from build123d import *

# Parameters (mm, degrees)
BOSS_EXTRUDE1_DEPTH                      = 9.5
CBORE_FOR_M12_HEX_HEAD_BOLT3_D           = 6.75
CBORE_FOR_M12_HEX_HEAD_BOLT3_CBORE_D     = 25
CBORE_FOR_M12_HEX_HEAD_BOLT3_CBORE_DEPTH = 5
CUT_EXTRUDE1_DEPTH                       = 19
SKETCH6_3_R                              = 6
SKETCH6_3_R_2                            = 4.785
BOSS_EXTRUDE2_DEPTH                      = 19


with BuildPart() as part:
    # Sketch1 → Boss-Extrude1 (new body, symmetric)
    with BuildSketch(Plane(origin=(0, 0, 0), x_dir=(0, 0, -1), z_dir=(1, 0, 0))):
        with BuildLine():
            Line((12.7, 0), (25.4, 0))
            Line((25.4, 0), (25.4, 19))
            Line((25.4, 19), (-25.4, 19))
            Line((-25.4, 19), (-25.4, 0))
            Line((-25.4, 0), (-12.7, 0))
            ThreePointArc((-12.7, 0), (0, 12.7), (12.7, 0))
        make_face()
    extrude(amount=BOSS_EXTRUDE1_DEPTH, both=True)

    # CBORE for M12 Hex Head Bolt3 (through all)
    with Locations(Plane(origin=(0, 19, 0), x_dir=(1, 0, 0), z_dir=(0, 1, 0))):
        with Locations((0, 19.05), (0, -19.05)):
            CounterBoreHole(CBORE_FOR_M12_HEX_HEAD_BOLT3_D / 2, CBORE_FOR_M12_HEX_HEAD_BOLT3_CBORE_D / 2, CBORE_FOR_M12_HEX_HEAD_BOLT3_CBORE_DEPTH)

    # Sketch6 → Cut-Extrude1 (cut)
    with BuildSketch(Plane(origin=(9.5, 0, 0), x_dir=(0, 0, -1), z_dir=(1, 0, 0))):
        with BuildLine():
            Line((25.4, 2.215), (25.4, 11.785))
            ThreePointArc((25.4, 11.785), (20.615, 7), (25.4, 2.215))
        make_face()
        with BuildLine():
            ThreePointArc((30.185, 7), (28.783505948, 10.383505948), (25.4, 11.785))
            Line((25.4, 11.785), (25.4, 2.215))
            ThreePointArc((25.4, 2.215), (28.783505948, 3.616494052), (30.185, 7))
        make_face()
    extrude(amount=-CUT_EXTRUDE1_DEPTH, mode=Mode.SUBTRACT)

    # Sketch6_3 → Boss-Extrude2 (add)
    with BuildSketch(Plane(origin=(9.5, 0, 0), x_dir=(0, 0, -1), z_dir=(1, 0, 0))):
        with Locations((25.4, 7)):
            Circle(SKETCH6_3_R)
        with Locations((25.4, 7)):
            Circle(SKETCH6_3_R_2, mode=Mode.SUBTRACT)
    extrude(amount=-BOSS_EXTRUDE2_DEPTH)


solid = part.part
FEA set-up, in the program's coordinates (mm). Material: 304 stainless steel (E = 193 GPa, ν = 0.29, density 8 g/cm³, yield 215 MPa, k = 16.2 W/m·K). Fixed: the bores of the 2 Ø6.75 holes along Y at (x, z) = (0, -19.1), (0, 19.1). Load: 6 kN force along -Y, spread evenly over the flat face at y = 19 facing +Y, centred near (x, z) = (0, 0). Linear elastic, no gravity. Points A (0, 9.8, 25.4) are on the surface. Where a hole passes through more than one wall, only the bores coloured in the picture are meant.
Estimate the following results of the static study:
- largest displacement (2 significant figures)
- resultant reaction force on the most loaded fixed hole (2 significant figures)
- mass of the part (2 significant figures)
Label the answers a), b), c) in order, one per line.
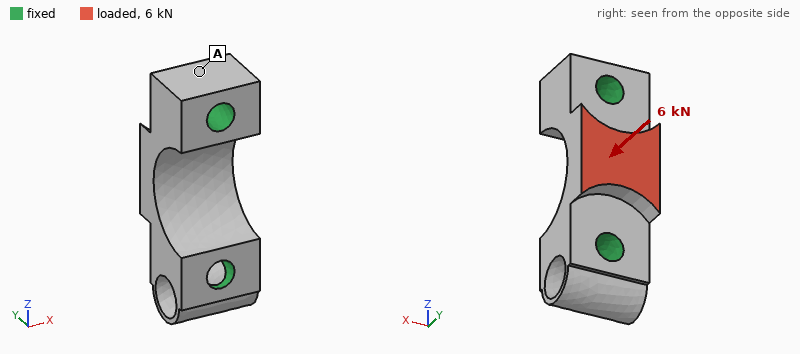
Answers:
a) 7.7 µm
b) 3.9 kN
c) 72 g
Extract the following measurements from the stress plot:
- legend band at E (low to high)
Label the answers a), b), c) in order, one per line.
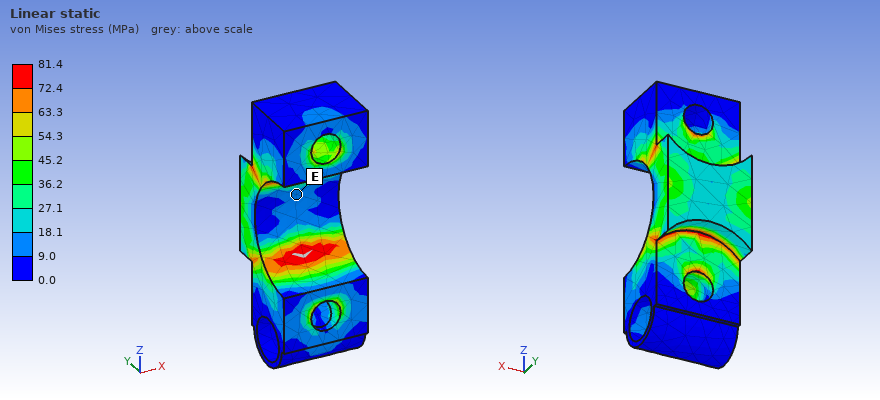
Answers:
a) 9.0 to 18.1 MPa
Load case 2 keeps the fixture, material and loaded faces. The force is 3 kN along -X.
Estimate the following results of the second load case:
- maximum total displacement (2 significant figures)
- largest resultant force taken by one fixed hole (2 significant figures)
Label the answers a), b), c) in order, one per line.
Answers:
a) 14 µm
b) 1.5 kN
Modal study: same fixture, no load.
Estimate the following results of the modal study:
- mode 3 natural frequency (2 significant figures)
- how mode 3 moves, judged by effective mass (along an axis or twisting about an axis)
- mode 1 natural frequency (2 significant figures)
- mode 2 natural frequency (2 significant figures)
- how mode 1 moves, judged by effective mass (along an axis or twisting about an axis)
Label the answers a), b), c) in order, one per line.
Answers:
a) 34 kHz
b) along Y
c) 23 kHz
d) 27 kHz
e) along X
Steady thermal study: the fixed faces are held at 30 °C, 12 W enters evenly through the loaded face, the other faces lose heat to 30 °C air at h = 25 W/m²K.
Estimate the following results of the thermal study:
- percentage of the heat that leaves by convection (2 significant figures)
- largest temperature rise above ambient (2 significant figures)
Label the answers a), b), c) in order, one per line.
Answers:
a) 9.9 %
b) 55 K
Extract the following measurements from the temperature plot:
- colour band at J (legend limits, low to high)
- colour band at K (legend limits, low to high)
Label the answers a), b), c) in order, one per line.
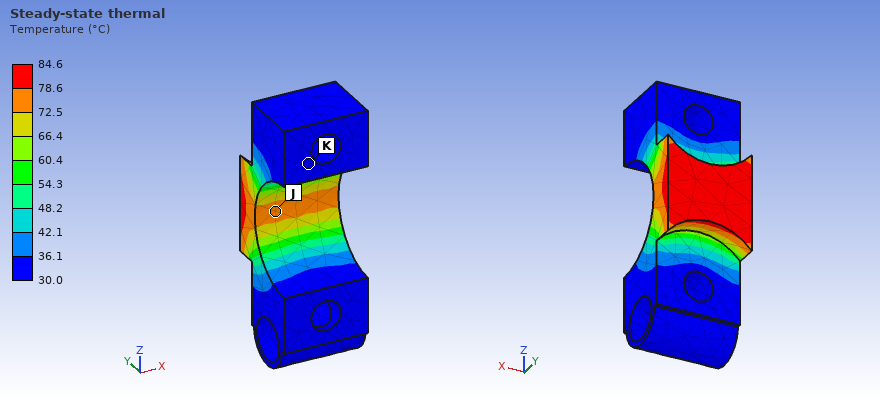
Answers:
a) 72.5 to 78.6 °C
b) 30.0 to 36.1 °C
